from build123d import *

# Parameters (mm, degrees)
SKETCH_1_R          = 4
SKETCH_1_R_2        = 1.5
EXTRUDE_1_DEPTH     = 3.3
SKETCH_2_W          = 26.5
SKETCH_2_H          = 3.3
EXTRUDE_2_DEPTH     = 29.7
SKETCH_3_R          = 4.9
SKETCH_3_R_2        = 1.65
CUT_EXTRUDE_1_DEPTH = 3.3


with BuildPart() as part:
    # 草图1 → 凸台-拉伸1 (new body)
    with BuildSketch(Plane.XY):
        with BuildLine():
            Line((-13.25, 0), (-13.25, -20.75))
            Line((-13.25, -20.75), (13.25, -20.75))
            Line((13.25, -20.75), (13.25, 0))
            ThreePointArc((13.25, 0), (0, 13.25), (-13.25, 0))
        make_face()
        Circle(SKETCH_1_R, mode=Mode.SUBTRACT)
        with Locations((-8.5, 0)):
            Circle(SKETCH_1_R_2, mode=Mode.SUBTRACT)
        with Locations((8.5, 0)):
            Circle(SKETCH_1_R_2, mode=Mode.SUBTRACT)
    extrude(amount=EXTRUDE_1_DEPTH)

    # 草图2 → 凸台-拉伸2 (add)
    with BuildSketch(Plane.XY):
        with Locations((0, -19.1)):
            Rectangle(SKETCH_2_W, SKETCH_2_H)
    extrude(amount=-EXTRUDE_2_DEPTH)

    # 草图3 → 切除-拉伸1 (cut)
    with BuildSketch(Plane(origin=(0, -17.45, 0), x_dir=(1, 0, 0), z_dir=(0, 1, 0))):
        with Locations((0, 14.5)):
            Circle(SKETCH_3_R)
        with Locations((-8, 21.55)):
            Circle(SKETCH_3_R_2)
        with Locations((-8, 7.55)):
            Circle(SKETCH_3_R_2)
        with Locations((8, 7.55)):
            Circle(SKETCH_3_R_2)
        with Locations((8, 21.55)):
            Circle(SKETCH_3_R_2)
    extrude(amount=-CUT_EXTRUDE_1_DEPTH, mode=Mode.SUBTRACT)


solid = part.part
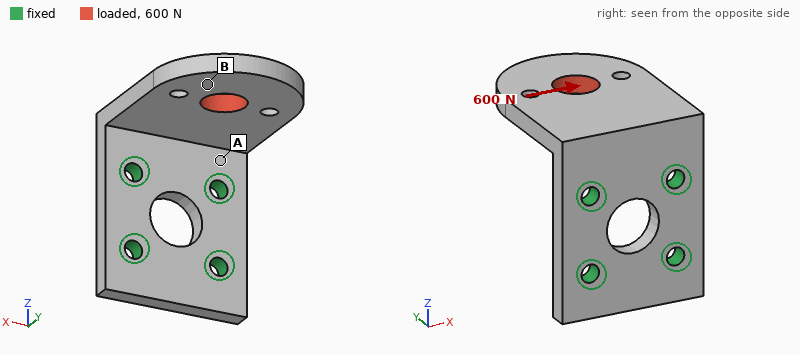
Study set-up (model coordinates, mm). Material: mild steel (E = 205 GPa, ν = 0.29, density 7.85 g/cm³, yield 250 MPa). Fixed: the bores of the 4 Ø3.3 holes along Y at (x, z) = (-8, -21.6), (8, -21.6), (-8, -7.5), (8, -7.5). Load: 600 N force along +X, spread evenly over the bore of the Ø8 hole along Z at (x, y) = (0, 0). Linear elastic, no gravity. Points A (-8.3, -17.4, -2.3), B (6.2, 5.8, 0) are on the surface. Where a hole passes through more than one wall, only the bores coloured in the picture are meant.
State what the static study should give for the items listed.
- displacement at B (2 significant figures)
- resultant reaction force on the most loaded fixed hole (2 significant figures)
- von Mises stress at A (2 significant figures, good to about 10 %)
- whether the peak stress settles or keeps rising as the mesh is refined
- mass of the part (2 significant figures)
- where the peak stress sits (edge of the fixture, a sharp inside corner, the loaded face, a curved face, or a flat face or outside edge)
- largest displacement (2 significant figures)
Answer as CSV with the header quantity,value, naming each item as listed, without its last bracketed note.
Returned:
quantity,value
displacement at B,37 µm
resultant reaction force on the most loaded fixed hole,750 N
von Mises stress at A,78 MPa
whether the peak stress settles or keeps rising as the mesh is refined,keeps rising
mass of the part,37 g
where the peak stress sits,edge of the fixture
largest displacement,45 µm
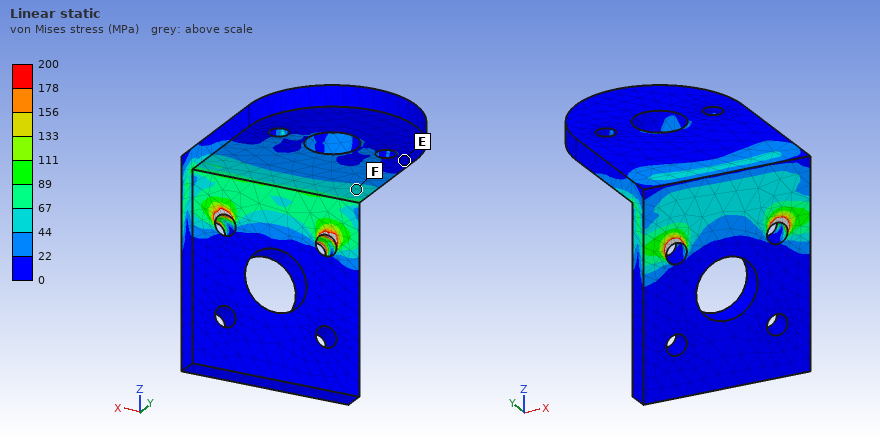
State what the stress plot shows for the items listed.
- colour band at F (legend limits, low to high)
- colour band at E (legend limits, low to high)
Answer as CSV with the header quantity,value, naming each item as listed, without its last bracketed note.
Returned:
quantity,value
colour band at F,44 to 67 MPa
colour band at E,0 to 22 MPa
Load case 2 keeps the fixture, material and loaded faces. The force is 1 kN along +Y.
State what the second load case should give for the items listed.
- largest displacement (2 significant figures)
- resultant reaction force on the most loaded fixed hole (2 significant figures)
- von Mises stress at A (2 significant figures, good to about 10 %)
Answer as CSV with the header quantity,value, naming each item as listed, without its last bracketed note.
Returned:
quantity,value
largest displacement,83 µm
resultant reaction force on the most loaded fixed hole,540 N
von Mises stress at A,85 MPa
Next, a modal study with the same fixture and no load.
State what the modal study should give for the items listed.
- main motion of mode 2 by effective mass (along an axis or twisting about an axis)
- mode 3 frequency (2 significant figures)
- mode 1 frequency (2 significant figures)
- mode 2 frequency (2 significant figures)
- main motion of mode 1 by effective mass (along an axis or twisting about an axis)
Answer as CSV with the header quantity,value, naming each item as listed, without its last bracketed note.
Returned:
quantity,value
main motion of mode 2 by effective mass,along X
mode 3 frequency,8600 Hz
mode 1 frequency,2200 Hz
mode 2 frequency,5500 Hz
main motion of mode 1 by effective mass,along Z
